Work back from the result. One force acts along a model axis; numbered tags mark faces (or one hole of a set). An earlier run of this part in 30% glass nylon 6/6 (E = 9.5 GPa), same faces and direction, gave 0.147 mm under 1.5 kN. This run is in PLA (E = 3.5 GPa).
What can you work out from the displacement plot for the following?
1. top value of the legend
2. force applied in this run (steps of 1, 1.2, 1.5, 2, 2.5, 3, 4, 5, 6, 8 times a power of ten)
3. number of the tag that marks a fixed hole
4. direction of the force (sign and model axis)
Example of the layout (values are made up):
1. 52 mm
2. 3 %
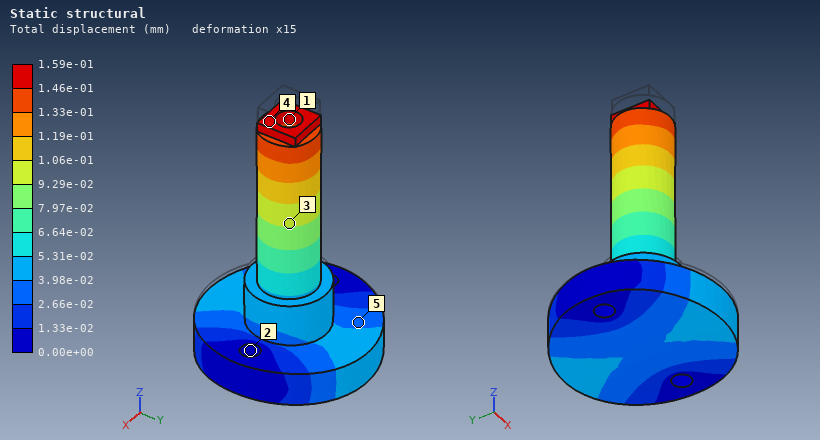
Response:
1. 1.59e-01 mm
2. 600 N
3. 2
4. -Z
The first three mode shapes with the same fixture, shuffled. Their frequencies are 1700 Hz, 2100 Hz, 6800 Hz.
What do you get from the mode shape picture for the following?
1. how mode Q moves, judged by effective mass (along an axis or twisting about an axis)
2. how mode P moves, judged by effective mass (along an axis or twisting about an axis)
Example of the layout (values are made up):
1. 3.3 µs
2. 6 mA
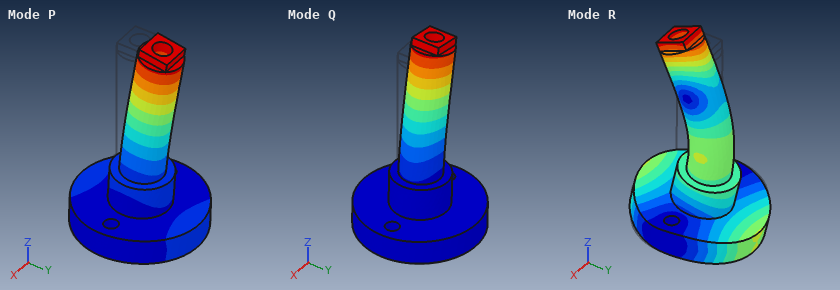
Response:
1. along X
2. along Y
